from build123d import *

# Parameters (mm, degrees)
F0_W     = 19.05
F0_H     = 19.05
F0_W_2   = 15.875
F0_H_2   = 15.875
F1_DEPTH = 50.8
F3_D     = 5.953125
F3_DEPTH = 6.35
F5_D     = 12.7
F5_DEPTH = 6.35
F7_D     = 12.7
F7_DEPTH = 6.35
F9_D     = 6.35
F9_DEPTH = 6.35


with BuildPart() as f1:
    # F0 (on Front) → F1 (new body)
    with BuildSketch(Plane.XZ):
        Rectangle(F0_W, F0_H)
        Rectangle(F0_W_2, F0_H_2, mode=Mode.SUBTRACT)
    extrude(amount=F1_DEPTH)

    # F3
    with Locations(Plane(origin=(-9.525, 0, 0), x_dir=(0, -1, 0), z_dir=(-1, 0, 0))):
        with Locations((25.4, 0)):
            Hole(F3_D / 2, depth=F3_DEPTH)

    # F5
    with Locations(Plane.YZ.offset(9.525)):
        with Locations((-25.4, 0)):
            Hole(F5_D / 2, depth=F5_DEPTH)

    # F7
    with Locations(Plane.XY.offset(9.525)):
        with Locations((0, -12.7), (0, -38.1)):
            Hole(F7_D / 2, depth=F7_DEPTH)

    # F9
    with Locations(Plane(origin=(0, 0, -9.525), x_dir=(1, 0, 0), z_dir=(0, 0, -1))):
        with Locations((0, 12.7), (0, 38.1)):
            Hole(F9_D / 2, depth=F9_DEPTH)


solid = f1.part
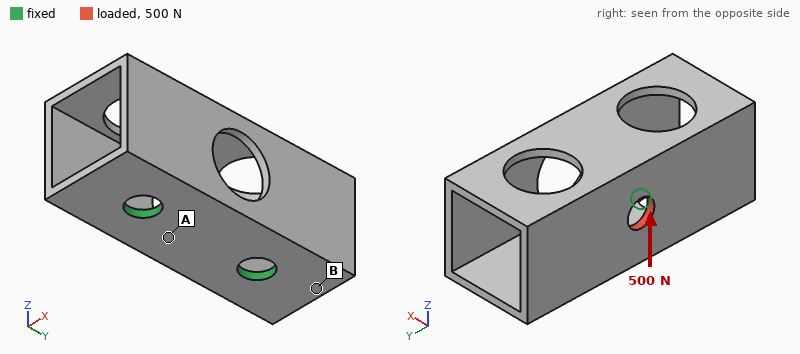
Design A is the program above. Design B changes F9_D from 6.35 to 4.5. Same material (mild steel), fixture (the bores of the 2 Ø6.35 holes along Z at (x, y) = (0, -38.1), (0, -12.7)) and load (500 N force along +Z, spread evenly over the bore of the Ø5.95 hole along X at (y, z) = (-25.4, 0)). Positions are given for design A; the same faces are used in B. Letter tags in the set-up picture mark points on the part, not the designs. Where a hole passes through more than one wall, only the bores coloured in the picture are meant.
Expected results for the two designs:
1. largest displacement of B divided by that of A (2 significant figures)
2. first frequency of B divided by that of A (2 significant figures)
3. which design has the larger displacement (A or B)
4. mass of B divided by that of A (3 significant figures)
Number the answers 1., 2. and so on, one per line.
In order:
1. 1.5
2. 0.89
3. B
4. 1.01
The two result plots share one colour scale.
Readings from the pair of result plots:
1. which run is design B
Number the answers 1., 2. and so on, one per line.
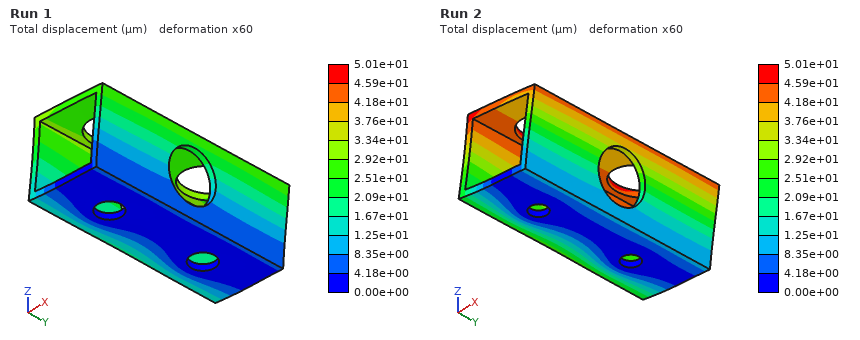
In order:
1. Run 2
